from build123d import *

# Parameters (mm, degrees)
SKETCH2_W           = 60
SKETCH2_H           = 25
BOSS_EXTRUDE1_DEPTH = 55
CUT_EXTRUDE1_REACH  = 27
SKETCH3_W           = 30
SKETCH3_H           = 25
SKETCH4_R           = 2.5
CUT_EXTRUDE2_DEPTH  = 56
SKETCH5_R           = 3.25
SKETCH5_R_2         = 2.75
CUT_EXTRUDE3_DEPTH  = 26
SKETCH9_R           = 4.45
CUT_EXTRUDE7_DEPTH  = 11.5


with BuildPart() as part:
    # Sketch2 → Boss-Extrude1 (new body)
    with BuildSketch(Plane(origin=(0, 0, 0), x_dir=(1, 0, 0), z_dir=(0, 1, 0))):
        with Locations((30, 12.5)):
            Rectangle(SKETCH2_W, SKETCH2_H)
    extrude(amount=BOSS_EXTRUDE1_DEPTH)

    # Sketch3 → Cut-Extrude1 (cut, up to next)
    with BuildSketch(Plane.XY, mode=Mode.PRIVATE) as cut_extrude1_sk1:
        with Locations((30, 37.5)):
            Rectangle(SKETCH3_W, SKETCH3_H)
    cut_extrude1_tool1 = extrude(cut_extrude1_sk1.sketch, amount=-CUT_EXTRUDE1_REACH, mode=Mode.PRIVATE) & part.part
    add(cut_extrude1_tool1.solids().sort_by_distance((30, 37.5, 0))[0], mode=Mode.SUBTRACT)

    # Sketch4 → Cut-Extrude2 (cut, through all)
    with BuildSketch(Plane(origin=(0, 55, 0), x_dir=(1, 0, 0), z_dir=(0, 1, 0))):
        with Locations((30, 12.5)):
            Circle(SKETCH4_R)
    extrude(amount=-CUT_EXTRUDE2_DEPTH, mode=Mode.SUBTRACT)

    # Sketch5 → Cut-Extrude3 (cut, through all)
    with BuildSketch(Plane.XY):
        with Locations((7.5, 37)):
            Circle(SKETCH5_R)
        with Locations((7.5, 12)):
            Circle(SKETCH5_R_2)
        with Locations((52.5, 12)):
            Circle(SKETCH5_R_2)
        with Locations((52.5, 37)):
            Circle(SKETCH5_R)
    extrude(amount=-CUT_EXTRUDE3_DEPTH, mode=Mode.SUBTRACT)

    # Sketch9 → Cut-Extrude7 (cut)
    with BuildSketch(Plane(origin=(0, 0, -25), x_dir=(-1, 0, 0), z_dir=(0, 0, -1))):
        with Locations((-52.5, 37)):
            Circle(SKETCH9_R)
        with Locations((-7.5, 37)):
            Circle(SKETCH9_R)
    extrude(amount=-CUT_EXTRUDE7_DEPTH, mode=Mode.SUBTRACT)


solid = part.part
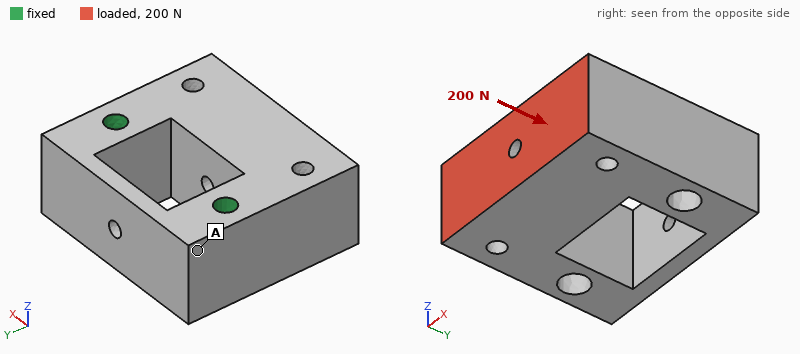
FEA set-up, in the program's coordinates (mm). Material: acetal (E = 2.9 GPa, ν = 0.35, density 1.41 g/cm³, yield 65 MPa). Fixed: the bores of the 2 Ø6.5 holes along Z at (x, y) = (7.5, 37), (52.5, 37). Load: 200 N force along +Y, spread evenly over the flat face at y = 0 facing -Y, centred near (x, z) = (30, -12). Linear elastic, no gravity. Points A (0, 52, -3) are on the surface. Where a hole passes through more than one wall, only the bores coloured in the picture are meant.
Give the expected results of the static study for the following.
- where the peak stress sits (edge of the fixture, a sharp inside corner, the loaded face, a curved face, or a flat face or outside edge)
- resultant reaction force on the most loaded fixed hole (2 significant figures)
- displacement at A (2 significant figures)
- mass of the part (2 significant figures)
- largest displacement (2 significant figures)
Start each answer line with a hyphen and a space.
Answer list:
- edge of the fixture
- 100 N
- 2.2 µm
- 84 g
- 12 µm
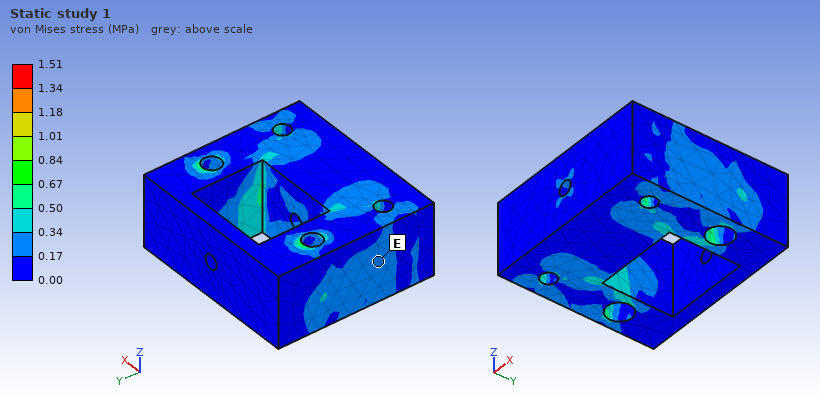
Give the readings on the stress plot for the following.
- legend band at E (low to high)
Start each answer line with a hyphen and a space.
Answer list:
- 0.17 to 0.34 MPa
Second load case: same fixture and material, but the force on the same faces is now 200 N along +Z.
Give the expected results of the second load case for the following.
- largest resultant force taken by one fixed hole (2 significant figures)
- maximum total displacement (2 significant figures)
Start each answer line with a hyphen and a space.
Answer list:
- 100 N
- 87 µm
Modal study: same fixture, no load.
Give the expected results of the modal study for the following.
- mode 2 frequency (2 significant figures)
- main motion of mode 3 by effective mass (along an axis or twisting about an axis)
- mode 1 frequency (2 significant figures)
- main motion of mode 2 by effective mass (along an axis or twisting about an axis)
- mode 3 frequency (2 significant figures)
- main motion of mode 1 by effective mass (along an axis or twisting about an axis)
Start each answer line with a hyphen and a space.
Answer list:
- 2800 Hz
- twisting about Y
- 1600 Hz
- along X
- 3200 Hz
- along Z
